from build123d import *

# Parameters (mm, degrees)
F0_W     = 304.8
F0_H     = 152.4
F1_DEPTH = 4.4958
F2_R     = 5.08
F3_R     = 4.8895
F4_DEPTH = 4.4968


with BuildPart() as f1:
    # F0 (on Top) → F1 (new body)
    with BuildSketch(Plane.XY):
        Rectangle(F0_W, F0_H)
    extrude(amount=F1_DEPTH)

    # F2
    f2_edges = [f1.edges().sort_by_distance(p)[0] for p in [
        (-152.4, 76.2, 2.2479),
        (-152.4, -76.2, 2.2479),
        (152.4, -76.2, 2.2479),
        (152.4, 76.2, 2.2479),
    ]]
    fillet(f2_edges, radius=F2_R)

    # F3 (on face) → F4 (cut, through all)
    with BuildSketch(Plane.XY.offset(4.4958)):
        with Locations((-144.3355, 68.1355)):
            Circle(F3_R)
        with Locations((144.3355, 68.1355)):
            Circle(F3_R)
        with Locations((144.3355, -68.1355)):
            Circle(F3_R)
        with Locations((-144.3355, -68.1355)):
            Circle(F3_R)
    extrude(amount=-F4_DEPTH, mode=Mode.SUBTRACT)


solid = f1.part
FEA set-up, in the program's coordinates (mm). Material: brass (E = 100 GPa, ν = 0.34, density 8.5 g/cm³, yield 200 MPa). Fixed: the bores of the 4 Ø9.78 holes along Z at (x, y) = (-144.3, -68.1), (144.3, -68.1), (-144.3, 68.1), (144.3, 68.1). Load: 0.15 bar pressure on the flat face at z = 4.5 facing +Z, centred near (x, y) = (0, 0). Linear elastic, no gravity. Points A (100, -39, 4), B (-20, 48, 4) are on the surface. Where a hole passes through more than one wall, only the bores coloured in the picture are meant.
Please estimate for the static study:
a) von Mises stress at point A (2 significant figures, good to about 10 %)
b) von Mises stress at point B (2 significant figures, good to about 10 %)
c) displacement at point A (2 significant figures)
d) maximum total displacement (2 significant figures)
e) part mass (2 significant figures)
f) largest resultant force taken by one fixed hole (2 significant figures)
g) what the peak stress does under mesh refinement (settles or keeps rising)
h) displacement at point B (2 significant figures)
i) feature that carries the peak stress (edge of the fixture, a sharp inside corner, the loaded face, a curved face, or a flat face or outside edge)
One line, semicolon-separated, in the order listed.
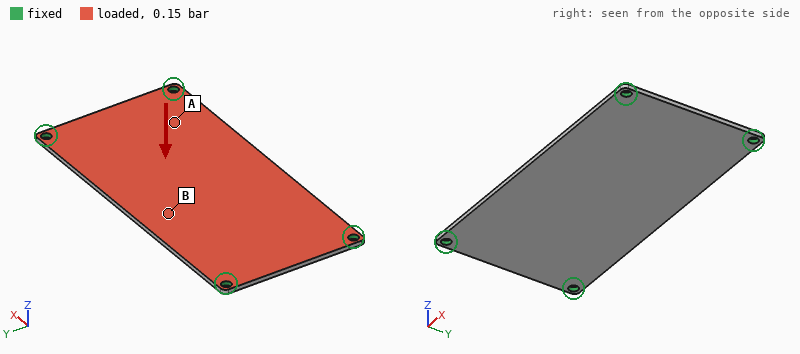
6.3 MPa; 17 MPa; 0.17 mm; 0.49 mm; 1.8 kg; 170 N; keeps rising; 0.46 mm; edge of the fixture
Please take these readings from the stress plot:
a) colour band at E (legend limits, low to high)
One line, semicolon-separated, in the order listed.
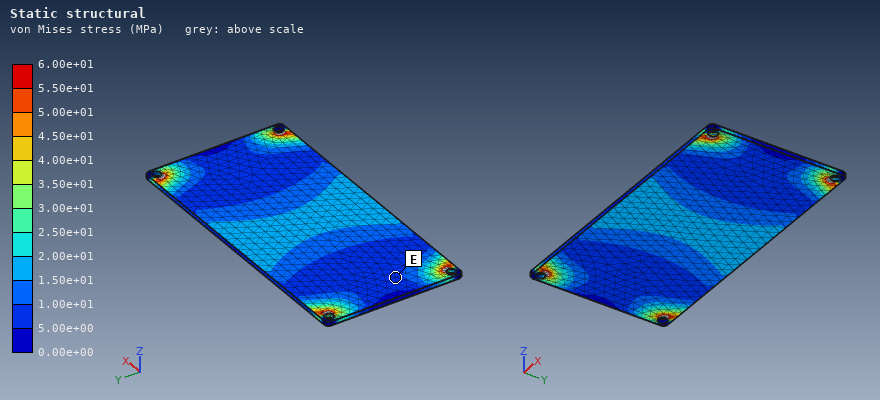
5.00e+00 to 1.00e+01 MPa
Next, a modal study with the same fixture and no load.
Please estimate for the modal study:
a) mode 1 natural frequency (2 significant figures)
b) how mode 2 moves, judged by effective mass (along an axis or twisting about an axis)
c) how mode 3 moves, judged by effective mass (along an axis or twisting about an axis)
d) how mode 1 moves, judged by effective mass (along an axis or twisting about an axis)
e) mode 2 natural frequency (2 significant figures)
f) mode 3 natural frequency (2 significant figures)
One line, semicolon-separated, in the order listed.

160 Hz; twisting about X; twisting about Y; along Z; 310 Hz; 460 Hz
